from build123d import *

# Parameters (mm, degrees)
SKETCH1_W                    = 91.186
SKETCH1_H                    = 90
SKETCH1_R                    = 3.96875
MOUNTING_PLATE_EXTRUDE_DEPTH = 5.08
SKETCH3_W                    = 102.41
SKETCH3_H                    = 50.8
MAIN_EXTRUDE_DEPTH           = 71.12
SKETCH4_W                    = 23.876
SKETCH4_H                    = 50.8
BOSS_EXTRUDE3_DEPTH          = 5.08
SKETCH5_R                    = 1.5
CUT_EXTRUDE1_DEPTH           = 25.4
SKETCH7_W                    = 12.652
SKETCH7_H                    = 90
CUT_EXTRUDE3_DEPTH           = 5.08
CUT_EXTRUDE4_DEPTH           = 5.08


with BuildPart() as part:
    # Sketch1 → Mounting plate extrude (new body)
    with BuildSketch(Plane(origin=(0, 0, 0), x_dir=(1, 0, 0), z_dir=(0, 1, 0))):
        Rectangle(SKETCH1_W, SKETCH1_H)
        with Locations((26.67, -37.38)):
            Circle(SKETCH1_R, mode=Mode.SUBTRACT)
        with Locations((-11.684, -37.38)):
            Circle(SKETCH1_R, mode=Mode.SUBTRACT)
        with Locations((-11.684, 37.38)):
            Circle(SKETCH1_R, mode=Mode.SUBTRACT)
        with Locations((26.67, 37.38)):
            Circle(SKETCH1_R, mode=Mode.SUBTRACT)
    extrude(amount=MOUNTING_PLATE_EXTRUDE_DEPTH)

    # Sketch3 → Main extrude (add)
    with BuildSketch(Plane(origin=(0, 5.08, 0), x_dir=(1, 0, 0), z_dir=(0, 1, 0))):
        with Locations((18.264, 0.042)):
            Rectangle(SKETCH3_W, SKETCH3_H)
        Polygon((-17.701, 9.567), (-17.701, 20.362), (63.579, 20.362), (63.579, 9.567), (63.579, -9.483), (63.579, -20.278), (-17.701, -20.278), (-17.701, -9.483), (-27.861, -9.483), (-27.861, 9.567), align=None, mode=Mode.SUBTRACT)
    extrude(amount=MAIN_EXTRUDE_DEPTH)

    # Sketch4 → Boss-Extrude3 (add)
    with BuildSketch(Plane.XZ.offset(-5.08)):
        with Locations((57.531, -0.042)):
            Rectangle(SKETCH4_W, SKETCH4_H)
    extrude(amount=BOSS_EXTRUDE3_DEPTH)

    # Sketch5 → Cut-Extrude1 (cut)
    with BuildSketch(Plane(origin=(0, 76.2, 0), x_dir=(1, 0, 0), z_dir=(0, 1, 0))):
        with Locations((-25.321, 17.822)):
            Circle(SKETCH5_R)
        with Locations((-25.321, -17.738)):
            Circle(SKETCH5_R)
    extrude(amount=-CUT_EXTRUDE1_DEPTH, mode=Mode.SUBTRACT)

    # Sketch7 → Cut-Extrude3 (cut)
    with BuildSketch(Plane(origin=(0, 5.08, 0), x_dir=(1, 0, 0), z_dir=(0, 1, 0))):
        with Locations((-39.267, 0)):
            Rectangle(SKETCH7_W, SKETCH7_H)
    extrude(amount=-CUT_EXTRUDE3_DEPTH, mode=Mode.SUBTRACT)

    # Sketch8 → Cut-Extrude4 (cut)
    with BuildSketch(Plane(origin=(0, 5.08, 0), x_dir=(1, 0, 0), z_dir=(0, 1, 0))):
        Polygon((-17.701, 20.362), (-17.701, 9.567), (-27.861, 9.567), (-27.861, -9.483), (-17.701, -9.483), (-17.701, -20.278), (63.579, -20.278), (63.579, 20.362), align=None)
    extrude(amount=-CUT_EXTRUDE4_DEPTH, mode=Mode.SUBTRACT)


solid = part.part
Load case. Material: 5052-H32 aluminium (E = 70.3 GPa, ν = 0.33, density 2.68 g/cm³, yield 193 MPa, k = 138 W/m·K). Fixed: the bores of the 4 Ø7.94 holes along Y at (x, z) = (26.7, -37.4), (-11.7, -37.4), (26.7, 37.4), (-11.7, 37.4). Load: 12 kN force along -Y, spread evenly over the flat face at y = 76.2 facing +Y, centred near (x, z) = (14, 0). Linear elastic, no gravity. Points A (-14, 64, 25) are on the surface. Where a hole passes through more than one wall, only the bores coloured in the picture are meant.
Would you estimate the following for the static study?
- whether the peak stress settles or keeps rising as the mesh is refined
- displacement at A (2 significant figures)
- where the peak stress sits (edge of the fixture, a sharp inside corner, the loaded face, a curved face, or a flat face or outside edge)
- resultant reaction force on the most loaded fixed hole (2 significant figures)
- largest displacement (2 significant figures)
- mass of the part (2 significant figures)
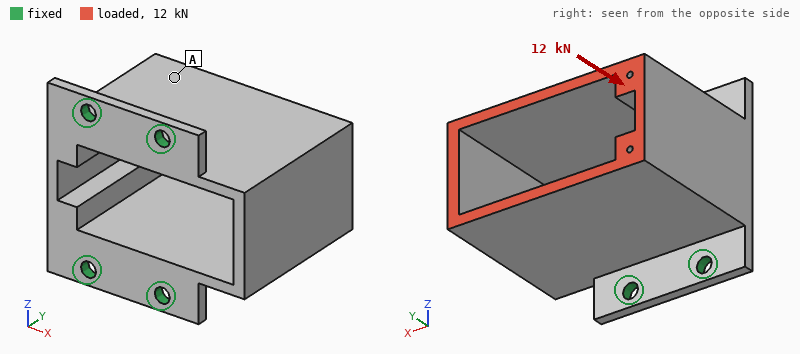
keeps rising
0.083 mm
edge of the fixture
3.9 kN
0.17 mm
390 g
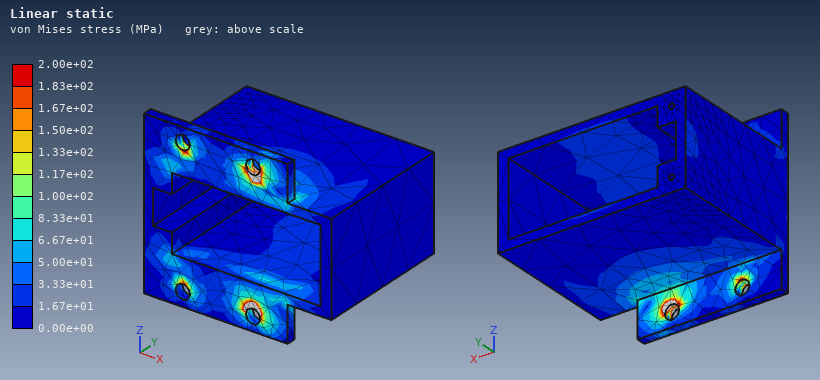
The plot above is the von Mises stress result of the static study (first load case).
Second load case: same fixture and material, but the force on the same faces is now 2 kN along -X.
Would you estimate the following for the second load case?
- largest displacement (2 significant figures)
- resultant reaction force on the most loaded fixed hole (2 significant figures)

0.16 mm
1.8 kN
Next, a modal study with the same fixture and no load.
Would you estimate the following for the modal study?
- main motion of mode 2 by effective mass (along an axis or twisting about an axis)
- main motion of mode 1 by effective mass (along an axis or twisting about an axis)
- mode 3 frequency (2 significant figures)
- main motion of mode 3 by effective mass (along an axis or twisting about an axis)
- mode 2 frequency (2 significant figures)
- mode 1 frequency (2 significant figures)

along Z
along X
2500 Hz
along Z
1800 Hz
1500 Hz
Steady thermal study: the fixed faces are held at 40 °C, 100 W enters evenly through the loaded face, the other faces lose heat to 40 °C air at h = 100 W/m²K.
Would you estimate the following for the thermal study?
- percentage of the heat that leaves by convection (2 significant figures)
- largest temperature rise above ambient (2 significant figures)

66 %
27 K
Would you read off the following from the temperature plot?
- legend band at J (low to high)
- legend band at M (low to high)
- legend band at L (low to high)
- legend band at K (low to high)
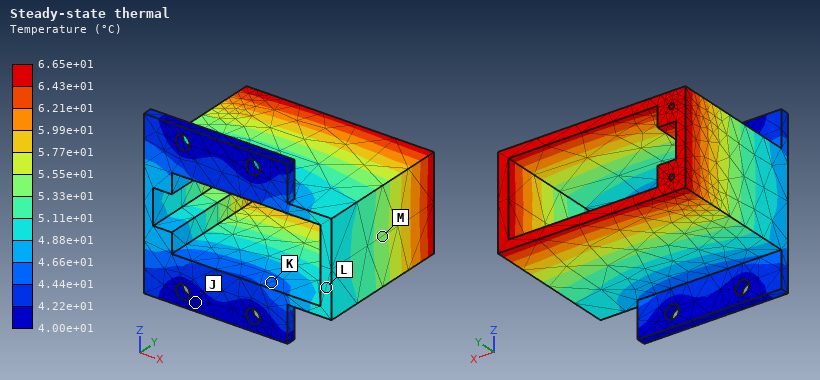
4.00e+01 to 4.22e+01 °C
5.33e+01 to 5.55e+01 °C
4.88e+01 to 5.11e+01 °C
4.44e+01 to 4.66e+01 °C
